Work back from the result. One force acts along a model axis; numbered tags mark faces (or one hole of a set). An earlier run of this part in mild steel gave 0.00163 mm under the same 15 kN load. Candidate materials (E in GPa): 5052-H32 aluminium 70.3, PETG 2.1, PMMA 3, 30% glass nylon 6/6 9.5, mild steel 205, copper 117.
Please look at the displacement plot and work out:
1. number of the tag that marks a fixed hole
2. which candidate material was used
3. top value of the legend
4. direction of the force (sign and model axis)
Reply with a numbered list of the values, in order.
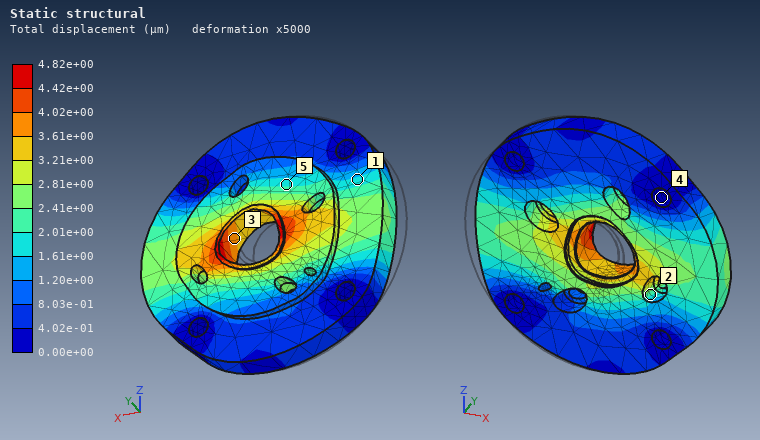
1. 4
2. 5052-H32 aluminium
3. 4.82e+00 µm
4. +X
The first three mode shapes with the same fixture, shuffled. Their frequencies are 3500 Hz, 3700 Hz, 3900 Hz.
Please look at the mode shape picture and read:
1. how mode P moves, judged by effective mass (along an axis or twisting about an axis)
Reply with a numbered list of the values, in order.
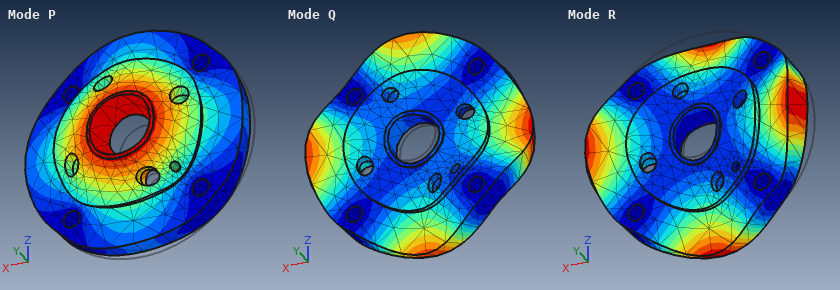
1. along Y
